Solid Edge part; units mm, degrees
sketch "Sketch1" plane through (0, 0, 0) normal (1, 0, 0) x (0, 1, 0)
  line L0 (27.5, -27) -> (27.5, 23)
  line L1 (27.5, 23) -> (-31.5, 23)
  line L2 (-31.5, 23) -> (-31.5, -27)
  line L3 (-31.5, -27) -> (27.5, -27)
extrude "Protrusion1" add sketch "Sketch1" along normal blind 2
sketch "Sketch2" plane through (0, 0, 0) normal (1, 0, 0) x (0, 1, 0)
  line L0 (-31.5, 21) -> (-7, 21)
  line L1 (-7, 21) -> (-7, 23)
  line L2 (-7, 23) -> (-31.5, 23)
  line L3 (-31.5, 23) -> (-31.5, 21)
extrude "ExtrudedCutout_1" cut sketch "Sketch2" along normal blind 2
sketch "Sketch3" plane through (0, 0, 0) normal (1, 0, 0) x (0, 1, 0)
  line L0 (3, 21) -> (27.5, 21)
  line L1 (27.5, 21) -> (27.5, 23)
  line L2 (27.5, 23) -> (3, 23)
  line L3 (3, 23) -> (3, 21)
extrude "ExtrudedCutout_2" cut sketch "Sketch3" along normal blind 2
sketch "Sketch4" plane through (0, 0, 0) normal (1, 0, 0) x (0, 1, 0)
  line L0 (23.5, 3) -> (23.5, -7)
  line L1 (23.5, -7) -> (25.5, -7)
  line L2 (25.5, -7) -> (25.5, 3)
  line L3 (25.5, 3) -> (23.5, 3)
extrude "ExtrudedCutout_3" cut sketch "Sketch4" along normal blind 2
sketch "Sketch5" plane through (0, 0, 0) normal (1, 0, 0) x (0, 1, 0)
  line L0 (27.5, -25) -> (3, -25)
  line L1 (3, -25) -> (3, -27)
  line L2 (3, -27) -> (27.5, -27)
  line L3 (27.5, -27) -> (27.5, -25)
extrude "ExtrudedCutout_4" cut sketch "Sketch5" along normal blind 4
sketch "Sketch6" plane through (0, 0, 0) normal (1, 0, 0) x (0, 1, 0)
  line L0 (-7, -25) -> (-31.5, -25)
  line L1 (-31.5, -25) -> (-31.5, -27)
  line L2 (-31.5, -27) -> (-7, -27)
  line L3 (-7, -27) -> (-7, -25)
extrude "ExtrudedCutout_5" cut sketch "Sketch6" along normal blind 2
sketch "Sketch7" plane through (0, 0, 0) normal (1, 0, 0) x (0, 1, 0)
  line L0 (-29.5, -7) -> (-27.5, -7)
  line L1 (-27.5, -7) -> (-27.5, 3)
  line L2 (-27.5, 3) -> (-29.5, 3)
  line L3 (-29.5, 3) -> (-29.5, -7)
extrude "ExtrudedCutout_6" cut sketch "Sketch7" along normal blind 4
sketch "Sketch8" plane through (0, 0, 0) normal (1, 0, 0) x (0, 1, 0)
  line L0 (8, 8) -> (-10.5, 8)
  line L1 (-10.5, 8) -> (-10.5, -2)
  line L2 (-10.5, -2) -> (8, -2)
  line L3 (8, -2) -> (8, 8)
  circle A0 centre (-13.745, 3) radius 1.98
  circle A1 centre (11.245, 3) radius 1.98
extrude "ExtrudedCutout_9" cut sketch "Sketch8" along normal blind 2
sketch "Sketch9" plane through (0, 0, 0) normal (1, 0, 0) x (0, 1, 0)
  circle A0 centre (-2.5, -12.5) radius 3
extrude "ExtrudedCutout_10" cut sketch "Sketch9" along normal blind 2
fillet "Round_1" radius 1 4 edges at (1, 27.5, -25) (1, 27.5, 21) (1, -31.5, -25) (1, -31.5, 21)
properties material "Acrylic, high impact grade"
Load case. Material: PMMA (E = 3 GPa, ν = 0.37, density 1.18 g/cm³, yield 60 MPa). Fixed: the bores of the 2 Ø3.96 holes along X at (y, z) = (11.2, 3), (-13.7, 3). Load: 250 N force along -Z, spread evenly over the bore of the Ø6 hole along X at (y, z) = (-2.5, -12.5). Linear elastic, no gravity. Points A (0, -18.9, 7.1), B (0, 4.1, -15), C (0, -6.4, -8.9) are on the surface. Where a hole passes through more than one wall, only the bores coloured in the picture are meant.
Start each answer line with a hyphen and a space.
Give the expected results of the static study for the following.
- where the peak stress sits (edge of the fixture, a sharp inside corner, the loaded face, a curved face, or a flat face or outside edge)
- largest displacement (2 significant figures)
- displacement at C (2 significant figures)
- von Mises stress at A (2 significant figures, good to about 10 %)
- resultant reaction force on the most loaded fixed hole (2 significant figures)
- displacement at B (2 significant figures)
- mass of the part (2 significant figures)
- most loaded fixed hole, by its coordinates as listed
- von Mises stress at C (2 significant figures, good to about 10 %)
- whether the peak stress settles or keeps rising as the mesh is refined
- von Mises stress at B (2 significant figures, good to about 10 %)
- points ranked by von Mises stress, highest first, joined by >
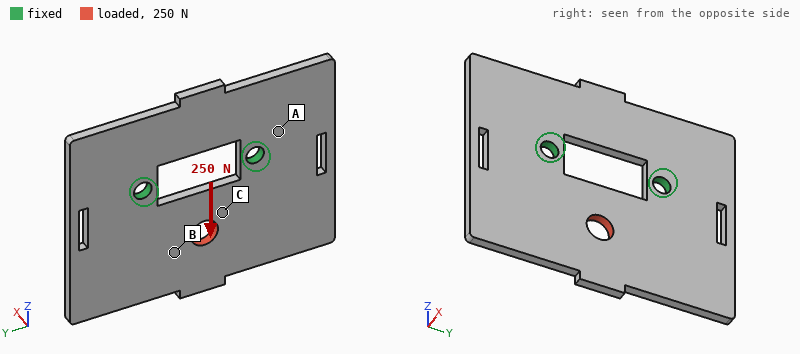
- a sharp inside corner
- 63 µm
- 48 µm
- 1.5 MPa
- 140 N
- 44 µm
- 5.8 g
- (-13.7, 3)
- 6.8 MPa
- keeps rising
- 4.8 MPa
- C > B > A
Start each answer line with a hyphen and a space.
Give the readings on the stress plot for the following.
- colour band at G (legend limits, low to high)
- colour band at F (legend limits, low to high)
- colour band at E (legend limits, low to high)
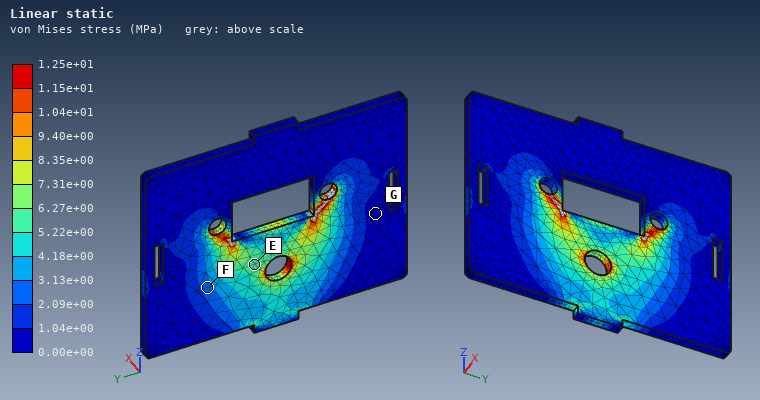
- 0.00e+00 to 1.04e+00 MPa
- 2.09e+00 to 3.13e+00 MPa
- 5.22e+00 to 6.27e+00 MPa
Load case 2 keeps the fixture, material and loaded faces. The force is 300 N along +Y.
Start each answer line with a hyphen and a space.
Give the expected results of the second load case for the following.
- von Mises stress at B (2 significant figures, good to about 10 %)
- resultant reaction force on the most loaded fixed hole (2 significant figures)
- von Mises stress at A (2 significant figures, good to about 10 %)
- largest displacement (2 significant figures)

- 6.9 MPa
- 210 N
- 3.4 MPa
- 0.19 mm
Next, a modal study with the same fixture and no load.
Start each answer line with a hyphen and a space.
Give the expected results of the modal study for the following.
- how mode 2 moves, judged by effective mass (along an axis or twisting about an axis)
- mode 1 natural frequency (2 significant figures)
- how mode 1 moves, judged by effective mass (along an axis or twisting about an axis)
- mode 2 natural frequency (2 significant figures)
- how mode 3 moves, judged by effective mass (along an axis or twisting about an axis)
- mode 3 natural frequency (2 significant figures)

- twisting about Z
- 530 Hz
- along X
- 810 Hz
- along X
- 1200 Hz
